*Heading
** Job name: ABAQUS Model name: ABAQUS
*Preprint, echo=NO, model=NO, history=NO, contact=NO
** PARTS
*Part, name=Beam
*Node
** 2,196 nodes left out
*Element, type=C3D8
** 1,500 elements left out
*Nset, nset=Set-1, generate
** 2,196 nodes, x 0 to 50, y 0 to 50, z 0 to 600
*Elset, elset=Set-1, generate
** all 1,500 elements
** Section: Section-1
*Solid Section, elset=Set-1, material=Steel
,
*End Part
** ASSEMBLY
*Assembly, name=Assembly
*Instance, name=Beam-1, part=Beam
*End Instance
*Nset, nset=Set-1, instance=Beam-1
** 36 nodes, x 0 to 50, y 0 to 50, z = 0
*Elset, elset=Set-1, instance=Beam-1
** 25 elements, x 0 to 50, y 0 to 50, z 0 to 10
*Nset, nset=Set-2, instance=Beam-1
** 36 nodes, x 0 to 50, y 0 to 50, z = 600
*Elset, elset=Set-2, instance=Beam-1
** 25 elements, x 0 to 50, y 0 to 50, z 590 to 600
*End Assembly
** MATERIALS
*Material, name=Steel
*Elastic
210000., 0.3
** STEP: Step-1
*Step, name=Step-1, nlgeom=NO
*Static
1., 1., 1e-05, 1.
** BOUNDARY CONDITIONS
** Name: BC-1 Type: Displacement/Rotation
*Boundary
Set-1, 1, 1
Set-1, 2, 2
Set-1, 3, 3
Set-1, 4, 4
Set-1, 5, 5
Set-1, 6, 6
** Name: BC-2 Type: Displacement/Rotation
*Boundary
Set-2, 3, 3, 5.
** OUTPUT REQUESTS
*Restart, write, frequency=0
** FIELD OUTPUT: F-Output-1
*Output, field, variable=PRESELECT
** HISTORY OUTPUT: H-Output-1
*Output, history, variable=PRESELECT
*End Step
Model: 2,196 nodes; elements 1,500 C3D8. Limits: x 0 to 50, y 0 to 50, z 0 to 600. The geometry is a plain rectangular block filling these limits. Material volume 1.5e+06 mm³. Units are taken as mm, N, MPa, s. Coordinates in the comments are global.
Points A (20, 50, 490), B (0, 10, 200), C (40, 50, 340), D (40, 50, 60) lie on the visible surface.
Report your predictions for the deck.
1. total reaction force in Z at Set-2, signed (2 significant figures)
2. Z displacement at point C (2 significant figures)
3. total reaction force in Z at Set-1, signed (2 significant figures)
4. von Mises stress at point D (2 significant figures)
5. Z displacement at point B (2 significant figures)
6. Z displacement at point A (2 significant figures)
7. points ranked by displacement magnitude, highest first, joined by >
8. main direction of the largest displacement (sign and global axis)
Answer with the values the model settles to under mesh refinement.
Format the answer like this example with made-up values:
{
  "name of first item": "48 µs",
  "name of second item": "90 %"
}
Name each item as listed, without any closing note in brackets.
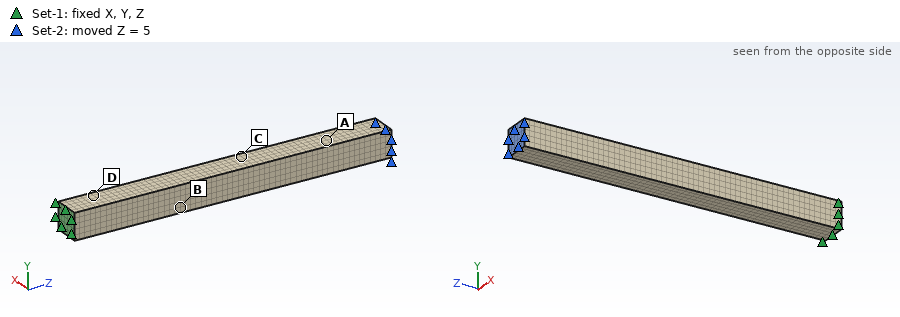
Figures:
{
  "total reaction force in Z at Set-2, signed": "4.4e+06 N",
  "Z displacement at point C": "2.8 mm",
  "total reaction force in Z at Set-1, signed": "-4.4e+06 N",
  "von Mises stress at point D": "1800 MPa",
  "Z displacement at point B": "1.7 mm",
  "Z displacement at point A": "4.1 mm",
  "points ranked by displacement magnitude, highest first, joined by >": "A > C > B > D",
  "main direction of the largest displacement": "+Z"
}
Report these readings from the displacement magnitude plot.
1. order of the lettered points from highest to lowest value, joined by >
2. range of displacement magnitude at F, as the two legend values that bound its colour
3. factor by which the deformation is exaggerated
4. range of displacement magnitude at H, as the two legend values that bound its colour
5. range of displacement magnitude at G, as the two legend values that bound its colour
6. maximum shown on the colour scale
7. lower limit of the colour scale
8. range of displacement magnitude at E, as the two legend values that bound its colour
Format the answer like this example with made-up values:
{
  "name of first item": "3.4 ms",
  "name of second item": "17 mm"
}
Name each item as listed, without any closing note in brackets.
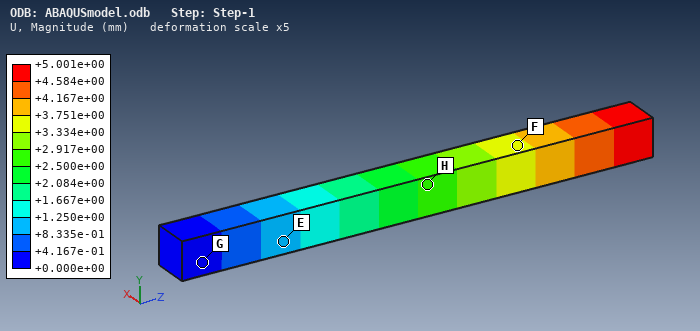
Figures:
{
  "order of the lettered points from highest to lowest value, joined by >": "F > H > E > G",
  "range of displacement magnitude at F, as the two legend values that bound its colour": "+3.334e+00 to +3.751e+00 mm",
  "factor by which the deformation is exaggerated": "5",
  "range of displacement magnitude at H, as the two legend values that bound its colour": "+2.500e+00 to +2.917e+00 mm",
  "range of displacement magnitude at G, as the two legend values that bound its colour": "+0.000e+00 to +4.167e-01 mm",
  "maximum shown on the colour scale": "+5.001e+00 mm",
  "lower limit of the colour scale": "+0.000e+00 mm",
  "range of displacement magnitude at E, as the two legend values that bound its colour": "+8.335e-01 to +1.250e+00 mm"
}
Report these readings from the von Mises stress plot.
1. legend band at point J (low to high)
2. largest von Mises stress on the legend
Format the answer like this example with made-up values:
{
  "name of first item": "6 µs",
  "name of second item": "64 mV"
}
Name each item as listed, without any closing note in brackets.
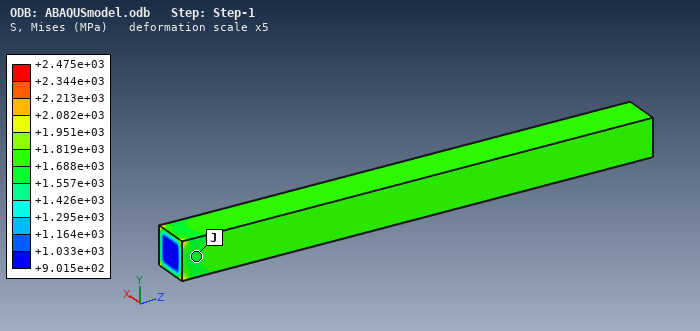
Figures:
{
  "legend band at point J": "+1.557e+03 to +1.688e+03 MPa",
  "largest von Mises stress on the legend": "+2.475e+03 MPa"
}
